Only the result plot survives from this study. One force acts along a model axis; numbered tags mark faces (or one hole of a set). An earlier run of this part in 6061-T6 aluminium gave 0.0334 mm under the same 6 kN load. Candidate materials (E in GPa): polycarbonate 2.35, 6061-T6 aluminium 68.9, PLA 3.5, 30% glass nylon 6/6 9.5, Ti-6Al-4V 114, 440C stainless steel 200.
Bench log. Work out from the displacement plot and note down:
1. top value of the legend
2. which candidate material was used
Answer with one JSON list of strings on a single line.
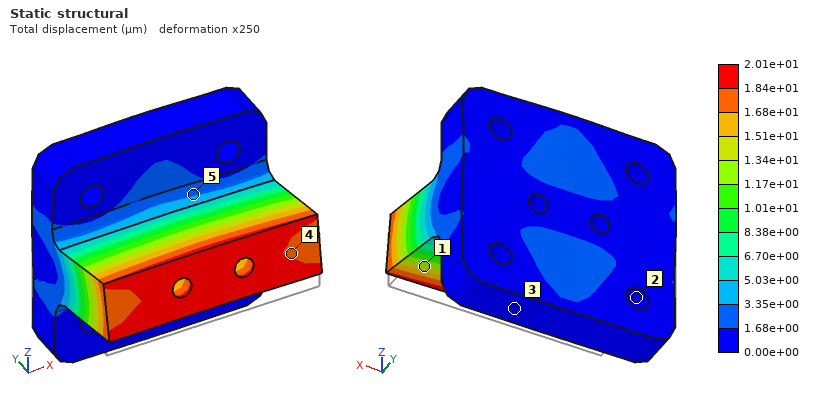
["2.01e+01 µm", "Ti-6Al-4V"]
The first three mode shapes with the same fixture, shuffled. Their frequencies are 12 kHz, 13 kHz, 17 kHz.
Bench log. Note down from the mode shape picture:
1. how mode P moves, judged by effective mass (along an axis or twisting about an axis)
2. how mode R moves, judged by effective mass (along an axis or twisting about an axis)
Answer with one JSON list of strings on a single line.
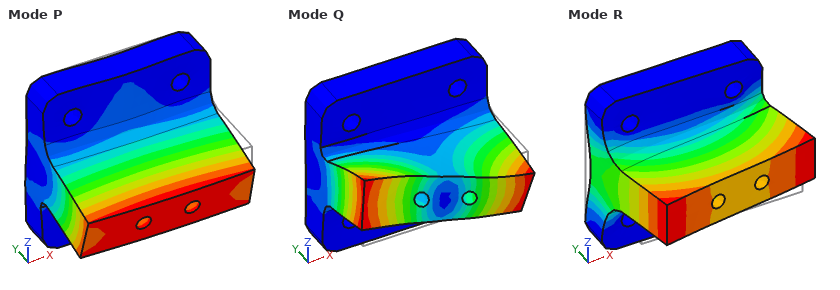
["along Z", "along X"]
